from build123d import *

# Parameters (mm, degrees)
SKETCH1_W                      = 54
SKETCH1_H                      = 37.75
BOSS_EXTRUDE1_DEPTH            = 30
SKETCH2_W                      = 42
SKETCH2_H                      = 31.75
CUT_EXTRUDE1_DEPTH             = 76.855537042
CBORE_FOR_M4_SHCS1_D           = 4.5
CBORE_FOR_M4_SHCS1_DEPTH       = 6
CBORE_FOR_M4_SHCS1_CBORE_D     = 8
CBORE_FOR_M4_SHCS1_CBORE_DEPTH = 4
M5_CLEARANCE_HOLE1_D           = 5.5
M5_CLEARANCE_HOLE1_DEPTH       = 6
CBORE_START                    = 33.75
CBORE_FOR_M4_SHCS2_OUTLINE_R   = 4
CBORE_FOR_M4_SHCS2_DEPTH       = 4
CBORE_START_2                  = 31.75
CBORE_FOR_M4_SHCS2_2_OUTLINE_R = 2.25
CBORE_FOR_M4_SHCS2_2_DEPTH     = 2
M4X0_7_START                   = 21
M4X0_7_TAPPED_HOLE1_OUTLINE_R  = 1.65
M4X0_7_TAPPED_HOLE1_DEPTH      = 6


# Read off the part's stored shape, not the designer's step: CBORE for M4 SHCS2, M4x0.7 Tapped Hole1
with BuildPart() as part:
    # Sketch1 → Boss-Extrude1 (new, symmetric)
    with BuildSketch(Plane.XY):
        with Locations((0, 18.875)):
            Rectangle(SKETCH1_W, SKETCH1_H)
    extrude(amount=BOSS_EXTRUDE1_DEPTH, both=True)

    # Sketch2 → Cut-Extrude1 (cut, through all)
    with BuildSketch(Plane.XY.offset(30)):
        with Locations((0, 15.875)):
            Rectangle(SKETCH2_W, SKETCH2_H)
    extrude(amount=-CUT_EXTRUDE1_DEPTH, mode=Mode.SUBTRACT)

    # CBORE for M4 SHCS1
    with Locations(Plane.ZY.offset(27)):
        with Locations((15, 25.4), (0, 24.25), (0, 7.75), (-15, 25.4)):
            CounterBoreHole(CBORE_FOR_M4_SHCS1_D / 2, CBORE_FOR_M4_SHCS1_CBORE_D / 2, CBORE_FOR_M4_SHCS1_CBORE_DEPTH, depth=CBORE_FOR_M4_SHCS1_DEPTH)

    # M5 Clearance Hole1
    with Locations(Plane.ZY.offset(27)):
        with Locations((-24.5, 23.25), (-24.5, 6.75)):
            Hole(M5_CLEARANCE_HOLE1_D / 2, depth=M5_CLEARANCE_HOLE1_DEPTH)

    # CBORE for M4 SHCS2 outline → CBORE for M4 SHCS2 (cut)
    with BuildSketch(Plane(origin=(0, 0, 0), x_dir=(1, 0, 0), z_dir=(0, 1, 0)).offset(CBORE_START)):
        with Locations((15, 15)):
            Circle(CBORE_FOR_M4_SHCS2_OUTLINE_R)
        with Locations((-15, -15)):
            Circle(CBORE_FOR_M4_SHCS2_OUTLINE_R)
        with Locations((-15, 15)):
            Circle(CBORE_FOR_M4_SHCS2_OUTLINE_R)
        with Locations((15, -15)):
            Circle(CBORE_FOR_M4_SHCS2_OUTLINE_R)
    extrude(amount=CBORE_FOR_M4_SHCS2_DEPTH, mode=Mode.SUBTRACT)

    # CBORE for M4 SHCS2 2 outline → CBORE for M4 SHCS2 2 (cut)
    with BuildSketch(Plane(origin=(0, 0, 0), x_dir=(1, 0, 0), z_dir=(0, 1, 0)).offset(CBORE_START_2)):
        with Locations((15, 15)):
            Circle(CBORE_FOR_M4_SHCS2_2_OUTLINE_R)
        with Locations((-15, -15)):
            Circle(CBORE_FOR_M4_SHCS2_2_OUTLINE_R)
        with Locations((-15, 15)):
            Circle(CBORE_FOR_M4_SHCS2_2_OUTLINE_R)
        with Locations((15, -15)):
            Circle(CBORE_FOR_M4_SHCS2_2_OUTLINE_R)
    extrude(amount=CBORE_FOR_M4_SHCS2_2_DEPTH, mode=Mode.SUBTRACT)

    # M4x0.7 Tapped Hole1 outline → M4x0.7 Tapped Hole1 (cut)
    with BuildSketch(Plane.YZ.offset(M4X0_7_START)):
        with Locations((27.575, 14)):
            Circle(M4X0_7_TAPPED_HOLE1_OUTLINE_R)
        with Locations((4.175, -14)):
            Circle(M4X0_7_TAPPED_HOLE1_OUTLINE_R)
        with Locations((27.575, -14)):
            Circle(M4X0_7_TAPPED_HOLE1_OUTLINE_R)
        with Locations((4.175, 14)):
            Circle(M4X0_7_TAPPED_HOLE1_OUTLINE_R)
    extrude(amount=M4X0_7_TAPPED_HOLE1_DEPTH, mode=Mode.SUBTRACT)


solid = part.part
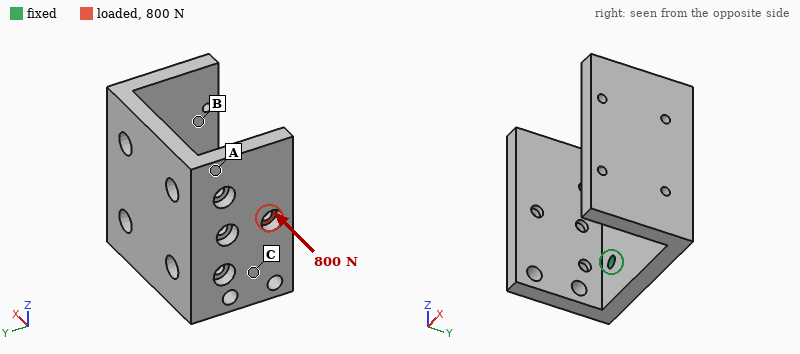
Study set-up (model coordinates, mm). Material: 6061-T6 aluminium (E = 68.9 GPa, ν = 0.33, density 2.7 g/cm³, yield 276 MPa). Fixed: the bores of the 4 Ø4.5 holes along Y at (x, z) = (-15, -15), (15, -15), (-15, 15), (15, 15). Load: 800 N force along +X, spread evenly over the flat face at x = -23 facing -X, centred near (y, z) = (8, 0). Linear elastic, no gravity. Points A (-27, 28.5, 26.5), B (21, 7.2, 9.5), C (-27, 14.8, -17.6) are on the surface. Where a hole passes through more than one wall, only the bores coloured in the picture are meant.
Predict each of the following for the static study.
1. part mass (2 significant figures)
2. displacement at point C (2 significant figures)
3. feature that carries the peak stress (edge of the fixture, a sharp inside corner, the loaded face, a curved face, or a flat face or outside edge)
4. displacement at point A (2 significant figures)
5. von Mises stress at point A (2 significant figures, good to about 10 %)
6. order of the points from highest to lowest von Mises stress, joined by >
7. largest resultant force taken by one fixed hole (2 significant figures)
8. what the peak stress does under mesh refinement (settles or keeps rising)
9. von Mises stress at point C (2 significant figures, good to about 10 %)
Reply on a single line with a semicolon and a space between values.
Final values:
110 g; 0.13 mm; edge of the fixture; 0.050 mm; 53 MPa; A > C > B; 1.1 kN; keeps rising; 22 MPa
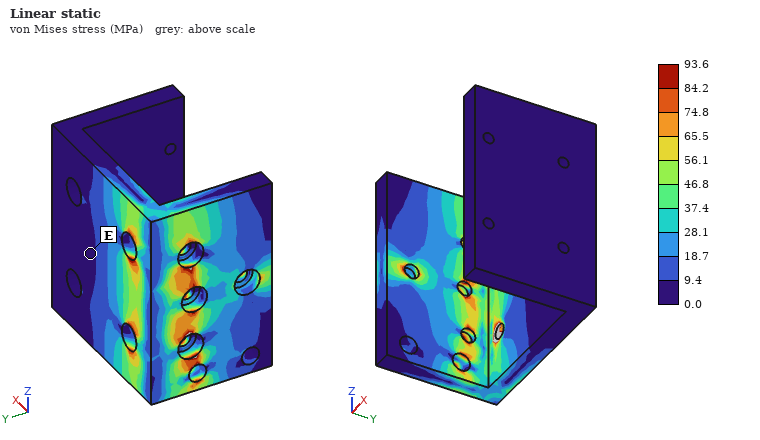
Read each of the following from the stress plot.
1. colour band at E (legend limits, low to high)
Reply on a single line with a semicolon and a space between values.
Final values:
0.0 to 9.4 MPa
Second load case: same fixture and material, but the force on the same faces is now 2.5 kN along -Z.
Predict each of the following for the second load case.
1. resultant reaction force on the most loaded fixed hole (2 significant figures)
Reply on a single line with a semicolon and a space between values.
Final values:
2.6 kN
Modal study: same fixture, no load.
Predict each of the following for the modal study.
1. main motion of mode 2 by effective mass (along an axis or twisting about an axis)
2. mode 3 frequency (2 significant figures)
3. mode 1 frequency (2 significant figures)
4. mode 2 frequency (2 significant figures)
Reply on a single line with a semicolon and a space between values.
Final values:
along X; 4700 Hz; 2500 Hz; 2600 Hz
